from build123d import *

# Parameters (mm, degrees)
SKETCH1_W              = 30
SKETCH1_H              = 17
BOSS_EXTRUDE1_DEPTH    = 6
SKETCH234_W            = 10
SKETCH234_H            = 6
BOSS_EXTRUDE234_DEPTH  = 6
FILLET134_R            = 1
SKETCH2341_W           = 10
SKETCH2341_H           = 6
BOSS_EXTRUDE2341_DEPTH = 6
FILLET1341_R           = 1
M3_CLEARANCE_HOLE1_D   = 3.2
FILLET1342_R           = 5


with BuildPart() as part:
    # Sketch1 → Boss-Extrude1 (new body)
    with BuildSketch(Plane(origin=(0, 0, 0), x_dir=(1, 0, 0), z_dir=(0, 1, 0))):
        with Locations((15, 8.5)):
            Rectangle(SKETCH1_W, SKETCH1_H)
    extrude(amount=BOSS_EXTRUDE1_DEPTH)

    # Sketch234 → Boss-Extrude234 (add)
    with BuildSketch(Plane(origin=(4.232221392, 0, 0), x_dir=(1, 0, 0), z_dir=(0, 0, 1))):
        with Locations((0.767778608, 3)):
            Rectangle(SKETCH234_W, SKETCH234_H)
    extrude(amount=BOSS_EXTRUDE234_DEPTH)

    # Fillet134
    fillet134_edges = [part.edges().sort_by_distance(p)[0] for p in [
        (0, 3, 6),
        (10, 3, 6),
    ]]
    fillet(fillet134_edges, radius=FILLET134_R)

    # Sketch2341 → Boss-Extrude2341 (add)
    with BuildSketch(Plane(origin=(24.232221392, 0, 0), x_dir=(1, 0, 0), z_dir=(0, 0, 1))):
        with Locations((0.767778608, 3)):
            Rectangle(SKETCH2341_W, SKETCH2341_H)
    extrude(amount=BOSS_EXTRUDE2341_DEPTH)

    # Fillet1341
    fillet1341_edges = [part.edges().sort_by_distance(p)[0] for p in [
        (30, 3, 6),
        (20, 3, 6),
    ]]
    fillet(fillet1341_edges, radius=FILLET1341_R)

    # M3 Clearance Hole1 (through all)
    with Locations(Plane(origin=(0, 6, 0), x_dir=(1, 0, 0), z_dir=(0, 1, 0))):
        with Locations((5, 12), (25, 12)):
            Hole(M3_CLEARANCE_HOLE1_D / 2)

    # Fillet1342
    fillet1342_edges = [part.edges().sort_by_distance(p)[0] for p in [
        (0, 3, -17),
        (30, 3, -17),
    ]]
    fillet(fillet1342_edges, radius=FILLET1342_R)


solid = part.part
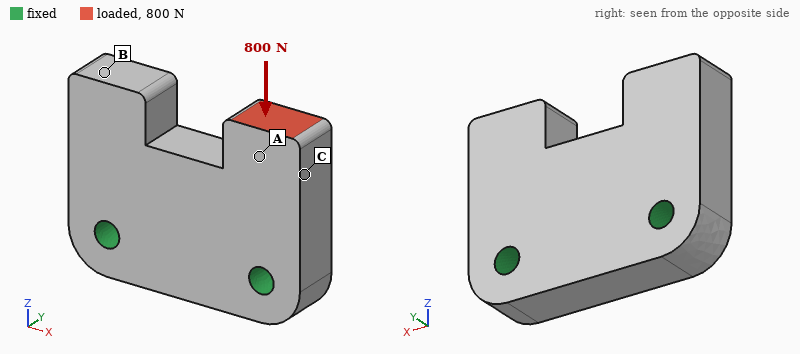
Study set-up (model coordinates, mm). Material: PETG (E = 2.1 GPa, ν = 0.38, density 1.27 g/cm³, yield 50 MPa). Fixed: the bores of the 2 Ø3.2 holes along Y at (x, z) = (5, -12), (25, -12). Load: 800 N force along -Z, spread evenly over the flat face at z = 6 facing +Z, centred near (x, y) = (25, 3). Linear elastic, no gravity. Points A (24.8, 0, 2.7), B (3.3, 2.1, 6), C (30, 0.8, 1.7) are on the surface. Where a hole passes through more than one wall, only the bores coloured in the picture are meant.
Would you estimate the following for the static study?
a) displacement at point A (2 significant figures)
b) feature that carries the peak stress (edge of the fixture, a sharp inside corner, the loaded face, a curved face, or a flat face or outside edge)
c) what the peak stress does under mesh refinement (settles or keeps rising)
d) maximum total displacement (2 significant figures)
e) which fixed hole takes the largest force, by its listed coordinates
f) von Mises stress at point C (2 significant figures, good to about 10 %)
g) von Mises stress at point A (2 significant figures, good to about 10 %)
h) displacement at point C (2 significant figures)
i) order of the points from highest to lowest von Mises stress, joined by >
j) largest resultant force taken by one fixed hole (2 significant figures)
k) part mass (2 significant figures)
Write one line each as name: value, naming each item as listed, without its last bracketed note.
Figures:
displacement at point A: 0.11 mm
feature that carries the peak stress: edge of the fixture
what the peak stress does under mesh refinement: keeps rising
maximum total displacement: 0.15 mm
which fixed hole takes the largest force, by its listed coordinates: (25, -12)
von Mises stress at point C: 11 MPa
von Mises stress at point A: 17 MPa
displacement at point C: 0.12 mm
order of the points from highest to lowest von Mises stress, joined by >: A > C > B
largest resultant force taken by one fixed hole: 780 N
part mass: 4.6 g
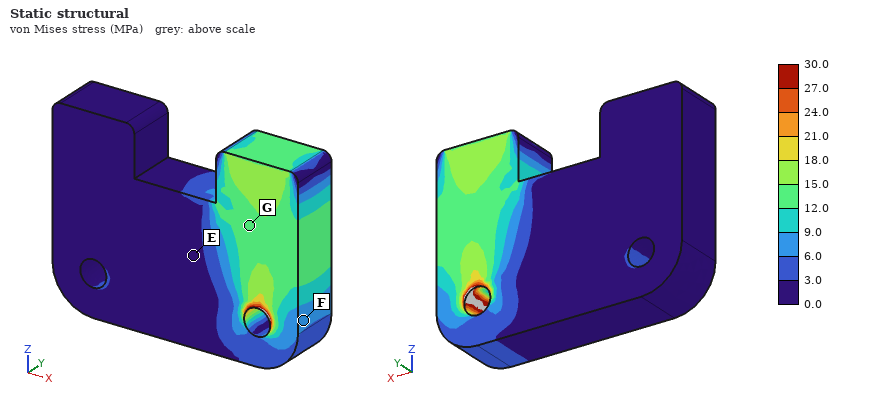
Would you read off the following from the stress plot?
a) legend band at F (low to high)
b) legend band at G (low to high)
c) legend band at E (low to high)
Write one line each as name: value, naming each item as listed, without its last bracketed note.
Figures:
legend band at F: 6.0 to 9.0 MPa
legend band at G: 12.0 to 15.0 MPa
legend band at E: 0.0 to 3.0 MPa
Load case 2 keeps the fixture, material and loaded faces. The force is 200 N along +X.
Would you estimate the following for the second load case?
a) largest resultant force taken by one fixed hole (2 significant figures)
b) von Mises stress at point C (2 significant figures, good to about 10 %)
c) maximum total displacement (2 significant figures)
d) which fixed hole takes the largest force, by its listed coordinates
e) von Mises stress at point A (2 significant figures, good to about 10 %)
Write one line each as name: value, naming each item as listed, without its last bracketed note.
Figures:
largest resultant force taken by one fixed hole: 220 N
von Mises stress at point C: 8.2 MPa
maximum total displacement: 0.18 mm
which fixed hole takes the largest force, by its listed coordinates: (5, -12)
von Mises stress at point A: 9.3 MPa
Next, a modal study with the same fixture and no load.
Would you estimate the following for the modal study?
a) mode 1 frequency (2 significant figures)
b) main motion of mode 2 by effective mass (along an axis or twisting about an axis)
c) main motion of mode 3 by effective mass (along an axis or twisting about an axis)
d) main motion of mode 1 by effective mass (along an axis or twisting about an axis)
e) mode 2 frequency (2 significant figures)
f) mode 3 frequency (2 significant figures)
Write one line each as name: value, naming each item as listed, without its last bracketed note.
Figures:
mode 1 frequency: 3800 Hz
main motion of mode 2 by effective mass: twisting about Z
main motion of mode 3 by effective mass: along X
main motion of mode 1 by effective mass: along Y
mode 2 frequency: 4800 Hz
mode 3 frequency: 8300 Hz
